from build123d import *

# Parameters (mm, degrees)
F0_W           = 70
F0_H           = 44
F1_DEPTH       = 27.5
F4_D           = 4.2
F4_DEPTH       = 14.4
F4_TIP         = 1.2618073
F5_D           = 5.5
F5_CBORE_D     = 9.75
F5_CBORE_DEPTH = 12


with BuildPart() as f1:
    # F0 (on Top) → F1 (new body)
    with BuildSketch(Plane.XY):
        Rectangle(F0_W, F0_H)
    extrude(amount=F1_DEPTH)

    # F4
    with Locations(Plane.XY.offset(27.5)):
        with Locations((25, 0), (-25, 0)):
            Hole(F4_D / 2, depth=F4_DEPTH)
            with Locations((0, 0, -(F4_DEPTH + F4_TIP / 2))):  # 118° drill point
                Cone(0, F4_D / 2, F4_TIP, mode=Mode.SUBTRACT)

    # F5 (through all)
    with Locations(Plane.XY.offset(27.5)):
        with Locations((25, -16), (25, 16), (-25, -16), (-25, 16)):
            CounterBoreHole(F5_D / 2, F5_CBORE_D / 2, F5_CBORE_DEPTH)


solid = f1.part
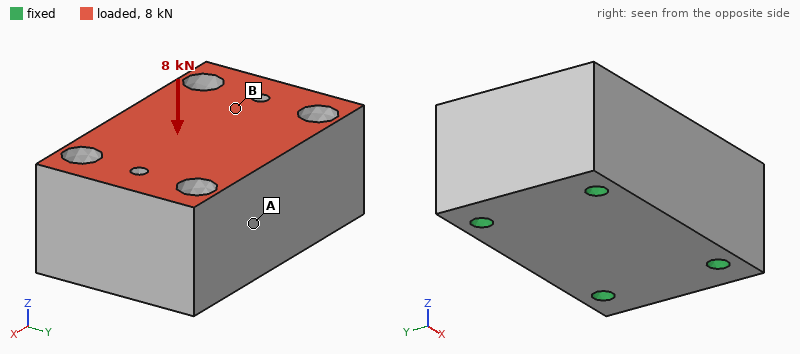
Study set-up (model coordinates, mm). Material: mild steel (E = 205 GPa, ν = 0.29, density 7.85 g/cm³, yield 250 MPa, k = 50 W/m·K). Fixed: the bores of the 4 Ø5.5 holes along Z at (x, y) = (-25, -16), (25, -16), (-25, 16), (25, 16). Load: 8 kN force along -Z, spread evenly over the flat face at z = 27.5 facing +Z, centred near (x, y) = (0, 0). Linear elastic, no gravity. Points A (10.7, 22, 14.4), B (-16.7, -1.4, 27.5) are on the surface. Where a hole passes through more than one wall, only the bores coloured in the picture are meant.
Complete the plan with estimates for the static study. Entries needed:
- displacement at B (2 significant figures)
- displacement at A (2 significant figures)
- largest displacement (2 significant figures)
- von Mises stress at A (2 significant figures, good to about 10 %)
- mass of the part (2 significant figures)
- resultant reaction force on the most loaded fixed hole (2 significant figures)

0.88 µm
0.83 µm
1.1 µm
4.0 MPa
620 g
2.1 kN
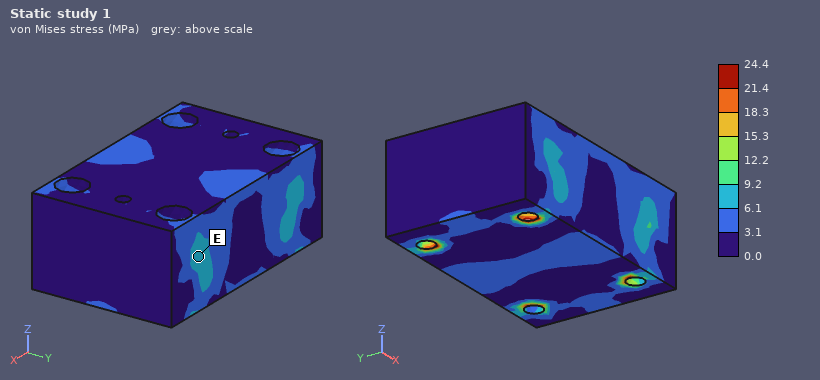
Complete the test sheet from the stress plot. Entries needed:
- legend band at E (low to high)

6.1 to 9.2 MPa
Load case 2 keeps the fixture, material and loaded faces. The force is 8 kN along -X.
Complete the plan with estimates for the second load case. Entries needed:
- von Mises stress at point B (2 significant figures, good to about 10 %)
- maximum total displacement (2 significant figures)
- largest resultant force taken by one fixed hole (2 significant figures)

5.8 MPa
2.1 µm
2.4 kN
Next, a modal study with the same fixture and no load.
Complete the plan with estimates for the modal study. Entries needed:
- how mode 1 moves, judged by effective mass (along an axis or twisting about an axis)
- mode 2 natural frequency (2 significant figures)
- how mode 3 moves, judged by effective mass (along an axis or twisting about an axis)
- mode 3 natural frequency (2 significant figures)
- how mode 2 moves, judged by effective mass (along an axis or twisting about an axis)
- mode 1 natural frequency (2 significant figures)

along Z
21 kHz
along X
26 kHz
along Y
20 kHz
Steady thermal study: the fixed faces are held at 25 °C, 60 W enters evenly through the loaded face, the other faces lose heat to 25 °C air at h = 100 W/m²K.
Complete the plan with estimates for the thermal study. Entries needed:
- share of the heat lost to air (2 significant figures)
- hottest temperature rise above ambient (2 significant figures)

10 %
13 K
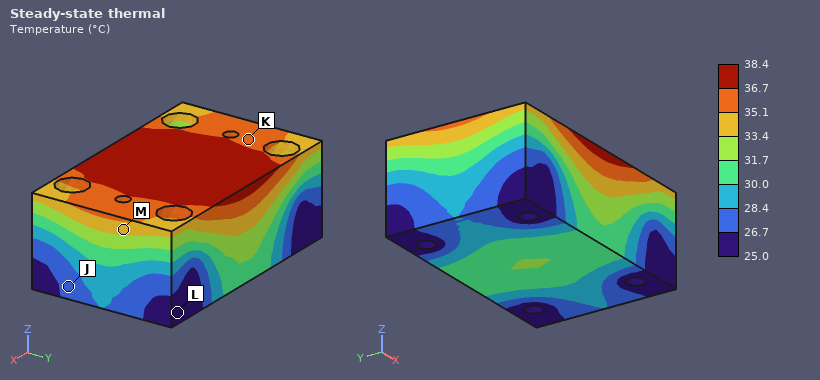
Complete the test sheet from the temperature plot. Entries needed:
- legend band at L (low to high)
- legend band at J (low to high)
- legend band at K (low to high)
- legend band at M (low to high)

25.0 to 26.7 °C
26.7 to 28.4 °C
35.1 to 36.7 °C
33.4 to 35.1 °C
